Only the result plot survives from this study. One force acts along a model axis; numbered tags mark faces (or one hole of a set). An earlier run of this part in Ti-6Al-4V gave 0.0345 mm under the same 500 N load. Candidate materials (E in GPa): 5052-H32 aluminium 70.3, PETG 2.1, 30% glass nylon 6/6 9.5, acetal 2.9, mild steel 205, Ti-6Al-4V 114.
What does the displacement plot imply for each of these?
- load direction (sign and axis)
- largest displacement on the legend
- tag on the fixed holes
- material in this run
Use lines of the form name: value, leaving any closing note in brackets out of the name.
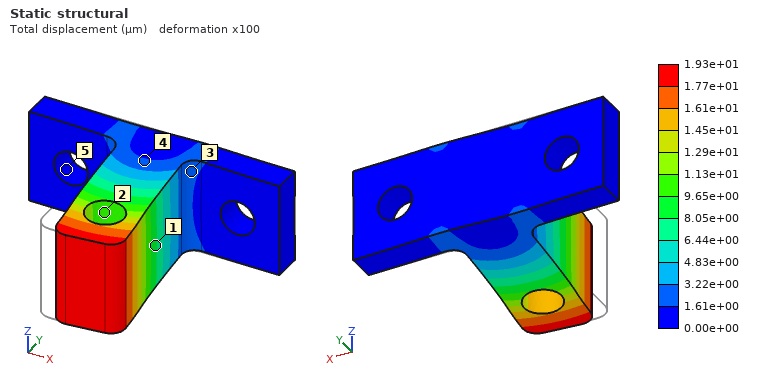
load direction: +X
largest displacement on the legend: 1.93e+01 µm
tag on the fixed holes: 5
material in this run: mild steel
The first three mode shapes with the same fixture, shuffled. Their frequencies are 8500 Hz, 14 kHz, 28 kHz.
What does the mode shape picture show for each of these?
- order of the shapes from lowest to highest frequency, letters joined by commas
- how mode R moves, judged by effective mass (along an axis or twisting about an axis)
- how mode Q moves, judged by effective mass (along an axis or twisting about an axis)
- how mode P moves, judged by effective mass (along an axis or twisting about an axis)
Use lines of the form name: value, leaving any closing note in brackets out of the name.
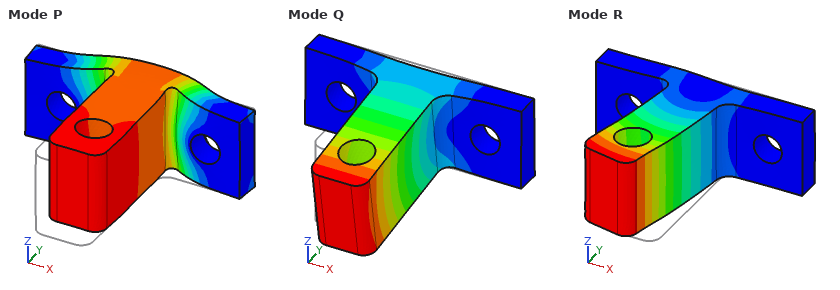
order of the shapes from lowest to highest frequency, letters joined by commas: Q, R, P
how mode R moves, judged by effective mass: along X
how mode Q moves, judged by effective mass: along Z
how mode P moves, judged by effective mass: along Y
